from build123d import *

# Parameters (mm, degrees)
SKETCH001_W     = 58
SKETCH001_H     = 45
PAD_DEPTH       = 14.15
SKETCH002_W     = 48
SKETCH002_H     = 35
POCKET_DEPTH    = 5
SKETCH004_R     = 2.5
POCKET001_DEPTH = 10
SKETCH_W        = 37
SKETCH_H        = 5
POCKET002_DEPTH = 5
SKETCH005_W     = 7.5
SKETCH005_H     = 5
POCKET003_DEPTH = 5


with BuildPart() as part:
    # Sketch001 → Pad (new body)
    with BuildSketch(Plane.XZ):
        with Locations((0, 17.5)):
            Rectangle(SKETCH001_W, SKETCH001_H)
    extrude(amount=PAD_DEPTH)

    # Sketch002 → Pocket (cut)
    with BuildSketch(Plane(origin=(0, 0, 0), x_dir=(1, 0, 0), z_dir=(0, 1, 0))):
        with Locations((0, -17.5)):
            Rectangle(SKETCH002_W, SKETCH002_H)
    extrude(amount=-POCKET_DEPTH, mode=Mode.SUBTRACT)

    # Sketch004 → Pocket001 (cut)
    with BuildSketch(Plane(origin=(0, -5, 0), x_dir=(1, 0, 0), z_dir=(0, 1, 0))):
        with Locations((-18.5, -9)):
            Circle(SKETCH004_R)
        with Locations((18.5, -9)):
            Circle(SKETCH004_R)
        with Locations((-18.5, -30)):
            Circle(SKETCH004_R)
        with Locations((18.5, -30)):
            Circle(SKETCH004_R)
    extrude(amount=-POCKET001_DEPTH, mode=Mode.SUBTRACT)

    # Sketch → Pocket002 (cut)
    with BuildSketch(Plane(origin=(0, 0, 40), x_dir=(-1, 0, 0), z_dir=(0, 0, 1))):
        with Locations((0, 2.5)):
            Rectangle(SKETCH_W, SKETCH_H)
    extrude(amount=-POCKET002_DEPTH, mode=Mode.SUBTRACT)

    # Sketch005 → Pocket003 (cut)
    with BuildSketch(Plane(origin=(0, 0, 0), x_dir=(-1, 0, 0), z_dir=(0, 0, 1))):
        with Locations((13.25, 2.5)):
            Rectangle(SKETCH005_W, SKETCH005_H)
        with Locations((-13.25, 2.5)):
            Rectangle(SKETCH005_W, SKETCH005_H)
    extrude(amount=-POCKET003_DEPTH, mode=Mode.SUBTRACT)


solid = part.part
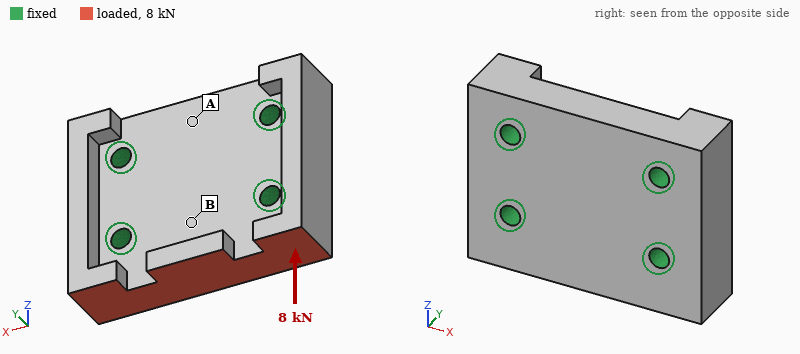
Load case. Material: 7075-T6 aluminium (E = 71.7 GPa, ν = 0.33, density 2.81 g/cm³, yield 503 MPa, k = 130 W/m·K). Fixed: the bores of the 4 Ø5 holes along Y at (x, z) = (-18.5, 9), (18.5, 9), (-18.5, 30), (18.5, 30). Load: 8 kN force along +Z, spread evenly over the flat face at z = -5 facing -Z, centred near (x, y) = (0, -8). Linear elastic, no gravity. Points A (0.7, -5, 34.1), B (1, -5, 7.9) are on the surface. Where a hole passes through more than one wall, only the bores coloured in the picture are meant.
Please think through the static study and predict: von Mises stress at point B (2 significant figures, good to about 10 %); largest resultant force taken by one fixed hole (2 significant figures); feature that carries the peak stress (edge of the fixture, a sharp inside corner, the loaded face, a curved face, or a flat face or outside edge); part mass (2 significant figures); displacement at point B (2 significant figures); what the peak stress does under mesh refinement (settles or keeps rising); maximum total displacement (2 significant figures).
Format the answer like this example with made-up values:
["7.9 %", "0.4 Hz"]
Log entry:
["20 MPa", "3.0 kN", "edge of the fixture", "75 g", "4.7 µm", "keeps rising", "19 µm"]
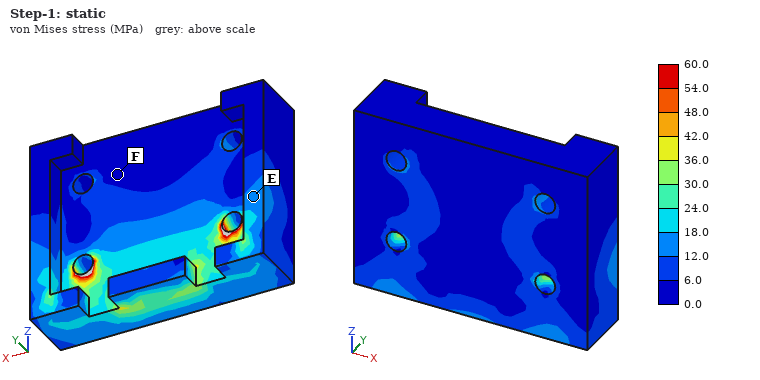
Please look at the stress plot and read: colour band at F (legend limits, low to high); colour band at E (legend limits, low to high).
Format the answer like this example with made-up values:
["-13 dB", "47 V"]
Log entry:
["0.0 to 6.0 MPa", "12.0 to 18.0 MPa"]
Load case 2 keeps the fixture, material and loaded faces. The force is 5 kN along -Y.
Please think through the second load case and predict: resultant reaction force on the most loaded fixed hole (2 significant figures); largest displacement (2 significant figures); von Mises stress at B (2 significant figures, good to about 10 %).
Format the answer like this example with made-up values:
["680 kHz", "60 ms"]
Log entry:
["3.1 kN", "42 µm", "35 MPa"]
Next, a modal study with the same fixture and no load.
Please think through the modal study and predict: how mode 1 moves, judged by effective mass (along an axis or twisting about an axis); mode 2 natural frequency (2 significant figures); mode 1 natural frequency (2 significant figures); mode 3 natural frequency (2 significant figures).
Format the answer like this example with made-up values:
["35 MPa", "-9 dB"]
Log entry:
["along Y", "25 kHz", "20 kHz", "26 kHz"]
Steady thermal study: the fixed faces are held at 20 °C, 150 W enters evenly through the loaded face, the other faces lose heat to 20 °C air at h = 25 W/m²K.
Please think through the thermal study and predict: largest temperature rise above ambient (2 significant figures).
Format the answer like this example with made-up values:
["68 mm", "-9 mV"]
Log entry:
["42 K"]
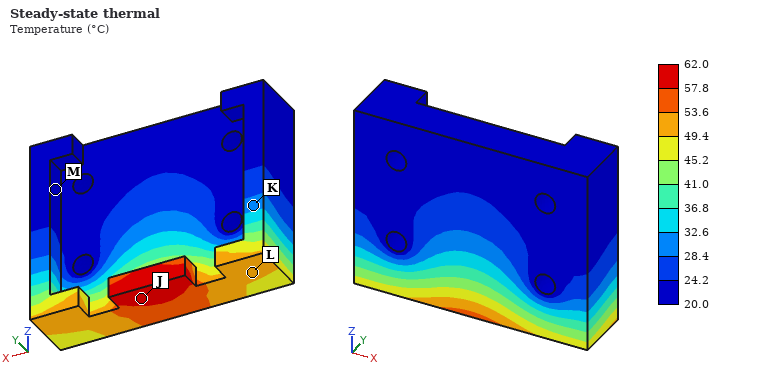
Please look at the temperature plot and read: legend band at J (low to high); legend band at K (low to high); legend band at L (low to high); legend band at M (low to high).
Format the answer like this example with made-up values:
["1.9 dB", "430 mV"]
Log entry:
["57.8 to 62.0 °C", "28.4 to 32.6 °C", "49.4 to 53.6 °C", "20.0 to 24.2 °C"]
